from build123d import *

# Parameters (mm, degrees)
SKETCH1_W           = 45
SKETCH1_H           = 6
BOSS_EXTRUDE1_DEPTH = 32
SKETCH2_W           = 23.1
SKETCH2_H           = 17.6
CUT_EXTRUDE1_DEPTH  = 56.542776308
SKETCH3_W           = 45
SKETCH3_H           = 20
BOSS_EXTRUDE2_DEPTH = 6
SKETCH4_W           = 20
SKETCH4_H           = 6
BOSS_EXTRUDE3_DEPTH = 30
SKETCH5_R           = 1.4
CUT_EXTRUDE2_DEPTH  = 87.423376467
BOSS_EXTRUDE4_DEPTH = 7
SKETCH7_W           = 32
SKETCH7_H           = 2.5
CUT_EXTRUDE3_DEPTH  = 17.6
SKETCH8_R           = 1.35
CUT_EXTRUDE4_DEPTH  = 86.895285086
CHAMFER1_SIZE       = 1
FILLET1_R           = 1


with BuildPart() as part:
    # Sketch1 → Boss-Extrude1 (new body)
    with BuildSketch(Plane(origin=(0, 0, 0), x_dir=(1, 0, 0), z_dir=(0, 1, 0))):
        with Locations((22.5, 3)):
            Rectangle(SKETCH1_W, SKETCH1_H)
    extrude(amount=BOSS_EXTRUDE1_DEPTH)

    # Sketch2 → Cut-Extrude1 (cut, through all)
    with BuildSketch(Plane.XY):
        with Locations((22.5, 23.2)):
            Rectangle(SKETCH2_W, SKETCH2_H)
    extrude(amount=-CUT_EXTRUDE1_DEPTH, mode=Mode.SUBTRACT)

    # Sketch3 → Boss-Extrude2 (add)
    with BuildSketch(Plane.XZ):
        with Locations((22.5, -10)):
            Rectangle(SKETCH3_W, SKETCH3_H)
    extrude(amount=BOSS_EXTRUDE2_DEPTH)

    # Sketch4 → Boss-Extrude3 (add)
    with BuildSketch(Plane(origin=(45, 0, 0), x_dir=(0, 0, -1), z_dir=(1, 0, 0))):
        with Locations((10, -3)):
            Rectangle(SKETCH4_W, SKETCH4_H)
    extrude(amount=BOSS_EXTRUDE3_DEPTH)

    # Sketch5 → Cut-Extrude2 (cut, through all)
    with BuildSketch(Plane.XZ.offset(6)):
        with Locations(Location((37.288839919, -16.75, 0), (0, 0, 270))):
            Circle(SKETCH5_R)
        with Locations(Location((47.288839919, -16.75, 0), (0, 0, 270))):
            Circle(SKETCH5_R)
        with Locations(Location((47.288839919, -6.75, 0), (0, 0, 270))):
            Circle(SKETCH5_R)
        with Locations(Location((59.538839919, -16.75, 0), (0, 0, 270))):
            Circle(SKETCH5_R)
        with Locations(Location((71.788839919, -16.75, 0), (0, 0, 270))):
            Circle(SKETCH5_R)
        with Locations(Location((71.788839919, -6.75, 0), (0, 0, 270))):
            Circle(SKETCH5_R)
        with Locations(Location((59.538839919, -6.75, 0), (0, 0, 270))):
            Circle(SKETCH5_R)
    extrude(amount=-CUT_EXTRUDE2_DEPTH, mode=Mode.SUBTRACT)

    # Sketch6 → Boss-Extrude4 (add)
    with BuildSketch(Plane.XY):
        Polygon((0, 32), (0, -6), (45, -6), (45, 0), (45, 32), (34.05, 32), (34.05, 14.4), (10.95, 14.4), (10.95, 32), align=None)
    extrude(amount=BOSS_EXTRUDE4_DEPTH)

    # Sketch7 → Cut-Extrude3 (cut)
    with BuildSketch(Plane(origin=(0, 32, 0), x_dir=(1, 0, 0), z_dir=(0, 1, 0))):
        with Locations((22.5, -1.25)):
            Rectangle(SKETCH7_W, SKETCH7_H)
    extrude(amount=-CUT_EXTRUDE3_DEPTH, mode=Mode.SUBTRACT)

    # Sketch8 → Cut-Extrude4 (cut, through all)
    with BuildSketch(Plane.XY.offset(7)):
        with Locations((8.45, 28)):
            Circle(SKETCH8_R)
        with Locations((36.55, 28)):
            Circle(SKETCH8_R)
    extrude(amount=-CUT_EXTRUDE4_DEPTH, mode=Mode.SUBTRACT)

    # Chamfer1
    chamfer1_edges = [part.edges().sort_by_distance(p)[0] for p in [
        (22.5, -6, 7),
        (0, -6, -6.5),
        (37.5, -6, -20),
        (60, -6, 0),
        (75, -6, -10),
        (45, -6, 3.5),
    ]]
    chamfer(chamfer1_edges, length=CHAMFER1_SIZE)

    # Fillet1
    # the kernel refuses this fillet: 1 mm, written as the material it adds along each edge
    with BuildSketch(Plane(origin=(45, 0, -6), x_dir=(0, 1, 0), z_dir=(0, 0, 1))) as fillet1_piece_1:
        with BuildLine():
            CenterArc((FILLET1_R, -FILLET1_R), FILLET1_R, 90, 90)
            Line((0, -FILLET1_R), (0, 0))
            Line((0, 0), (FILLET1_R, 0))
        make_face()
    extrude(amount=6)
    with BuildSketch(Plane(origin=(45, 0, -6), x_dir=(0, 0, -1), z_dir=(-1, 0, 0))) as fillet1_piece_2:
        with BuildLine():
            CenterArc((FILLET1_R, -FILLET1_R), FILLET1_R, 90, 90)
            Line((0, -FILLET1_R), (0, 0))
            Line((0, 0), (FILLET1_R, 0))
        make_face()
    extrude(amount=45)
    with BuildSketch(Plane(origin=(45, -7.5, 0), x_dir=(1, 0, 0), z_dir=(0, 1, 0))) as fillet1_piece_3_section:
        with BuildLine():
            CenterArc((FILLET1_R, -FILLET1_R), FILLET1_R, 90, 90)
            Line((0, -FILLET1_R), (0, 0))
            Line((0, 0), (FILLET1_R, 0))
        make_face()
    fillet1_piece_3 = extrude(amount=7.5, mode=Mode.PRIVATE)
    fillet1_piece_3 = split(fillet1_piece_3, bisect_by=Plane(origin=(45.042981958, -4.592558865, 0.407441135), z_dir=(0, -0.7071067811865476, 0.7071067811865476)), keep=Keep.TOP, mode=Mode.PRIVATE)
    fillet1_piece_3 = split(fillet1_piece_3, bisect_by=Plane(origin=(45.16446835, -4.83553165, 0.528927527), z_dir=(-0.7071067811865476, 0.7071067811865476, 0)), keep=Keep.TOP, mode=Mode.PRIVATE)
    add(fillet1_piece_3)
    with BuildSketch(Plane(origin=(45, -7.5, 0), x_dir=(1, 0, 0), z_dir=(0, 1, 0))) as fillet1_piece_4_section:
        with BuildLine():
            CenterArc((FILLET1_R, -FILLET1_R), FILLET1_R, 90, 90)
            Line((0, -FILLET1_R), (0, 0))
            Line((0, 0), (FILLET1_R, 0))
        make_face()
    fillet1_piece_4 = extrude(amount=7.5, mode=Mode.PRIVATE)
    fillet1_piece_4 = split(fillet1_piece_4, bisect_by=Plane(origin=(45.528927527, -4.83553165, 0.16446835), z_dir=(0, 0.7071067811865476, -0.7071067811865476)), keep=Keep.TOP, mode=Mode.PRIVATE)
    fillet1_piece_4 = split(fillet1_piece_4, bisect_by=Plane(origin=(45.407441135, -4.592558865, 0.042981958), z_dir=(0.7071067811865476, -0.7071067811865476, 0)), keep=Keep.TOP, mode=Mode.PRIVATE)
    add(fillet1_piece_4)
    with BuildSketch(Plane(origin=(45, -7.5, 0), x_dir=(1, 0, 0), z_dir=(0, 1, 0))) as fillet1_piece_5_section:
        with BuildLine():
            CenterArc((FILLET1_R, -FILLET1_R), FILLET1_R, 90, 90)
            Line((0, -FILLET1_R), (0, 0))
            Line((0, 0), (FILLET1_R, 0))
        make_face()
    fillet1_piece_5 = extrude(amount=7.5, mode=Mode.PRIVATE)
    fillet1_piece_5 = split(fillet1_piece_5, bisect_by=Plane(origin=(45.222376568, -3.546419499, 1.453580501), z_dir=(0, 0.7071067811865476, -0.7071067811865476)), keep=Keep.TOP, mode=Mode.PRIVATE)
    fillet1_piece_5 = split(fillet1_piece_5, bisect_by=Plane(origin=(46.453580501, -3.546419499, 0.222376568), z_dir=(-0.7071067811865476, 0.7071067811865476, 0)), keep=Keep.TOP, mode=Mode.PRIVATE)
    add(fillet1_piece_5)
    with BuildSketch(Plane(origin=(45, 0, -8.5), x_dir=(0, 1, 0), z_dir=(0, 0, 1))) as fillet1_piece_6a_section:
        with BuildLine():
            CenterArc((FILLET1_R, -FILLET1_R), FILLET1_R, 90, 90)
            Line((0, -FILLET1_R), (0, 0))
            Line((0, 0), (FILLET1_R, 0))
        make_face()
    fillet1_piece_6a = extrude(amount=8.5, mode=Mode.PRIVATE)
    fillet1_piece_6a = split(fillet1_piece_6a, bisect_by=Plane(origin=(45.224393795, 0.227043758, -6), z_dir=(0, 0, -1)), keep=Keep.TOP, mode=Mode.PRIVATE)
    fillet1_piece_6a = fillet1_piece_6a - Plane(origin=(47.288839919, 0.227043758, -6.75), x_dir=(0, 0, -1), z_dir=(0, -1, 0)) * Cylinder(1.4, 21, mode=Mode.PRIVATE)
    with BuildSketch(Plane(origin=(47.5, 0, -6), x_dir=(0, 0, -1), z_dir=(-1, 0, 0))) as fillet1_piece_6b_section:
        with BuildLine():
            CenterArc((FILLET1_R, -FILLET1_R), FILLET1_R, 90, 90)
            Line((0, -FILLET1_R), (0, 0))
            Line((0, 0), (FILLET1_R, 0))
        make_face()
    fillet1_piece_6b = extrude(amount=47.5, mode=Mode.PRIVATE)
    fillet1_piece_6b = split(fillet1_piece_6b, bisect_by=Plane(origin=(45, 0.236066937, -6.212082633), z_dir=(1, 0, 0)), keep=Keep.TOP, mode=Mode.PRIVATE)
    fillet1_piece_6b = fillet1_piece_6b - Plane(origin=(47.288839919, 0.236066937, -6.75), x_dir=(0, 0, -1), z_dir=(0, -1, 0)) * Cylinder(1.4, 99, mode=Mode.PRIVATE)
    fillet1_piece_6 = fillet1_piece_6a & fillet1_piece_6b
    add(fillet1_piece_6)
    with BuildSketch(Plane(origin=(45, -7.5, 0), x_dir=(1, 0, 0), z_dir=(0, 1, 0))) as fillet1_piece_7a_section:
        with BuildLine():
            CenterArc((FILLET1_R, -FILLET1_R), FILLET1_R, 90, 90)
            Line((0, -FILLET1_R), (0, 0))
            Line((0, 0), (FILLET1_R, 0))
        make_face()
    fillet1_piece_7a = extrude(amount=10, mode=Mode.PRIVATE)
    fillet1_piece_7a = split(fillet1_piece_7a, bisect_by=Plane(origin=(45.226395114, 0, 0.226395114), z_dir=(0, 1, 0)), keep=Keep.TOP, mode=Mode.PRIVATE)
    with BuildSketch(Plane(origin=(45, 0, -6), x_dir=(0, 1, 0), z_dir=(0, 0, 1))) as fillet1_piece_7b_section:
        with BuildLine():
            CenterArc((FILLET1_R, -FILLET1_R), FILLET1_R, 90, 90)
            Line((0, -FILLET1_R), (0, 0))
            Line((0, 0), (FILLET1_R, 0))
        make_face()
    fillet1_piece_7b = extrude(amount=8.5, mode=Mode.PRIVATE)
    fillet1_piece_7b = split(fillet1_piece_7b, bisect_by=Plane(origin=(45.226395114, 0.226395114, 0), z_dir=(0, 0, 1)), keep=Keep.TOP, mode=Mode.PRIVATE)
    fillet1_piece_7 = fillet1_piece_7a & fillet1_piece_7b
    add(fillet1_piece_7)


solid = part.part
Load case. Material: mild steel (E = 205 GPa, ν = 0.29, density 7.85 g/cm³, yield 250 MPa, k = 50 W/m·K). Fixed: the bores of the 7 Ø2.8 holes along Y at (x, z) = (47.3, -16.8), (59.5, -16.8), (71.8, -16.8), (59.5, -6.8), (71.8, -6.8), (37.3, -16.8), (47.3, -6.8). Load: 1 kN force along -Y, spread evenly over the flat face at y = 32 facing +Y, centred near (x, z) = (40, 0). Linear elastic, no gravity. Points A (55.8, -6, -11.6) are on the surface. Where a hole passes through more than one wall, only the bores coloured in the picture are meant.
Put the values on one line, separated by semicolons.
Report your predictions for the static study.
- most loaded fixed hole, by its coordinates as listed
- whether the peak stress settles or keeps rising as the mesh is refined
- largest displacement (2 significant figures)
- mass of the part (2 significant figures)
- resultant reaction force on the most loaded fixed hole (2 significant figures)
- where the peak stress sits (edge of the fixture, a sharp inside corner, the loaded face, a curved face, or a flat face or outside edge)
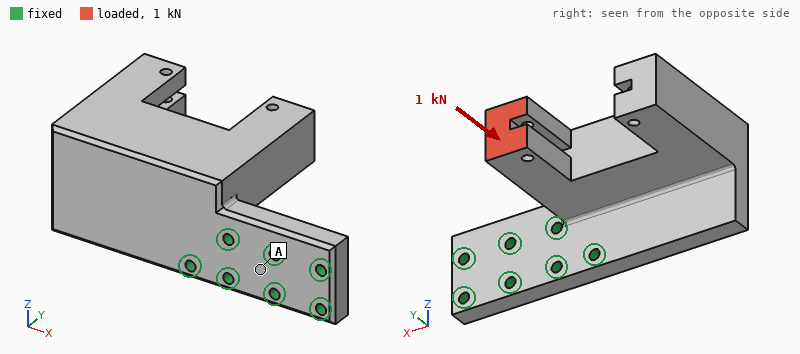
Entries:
(47.3, -6.8); keeps rising; 33 µm; 180 g; 1.0 kN; edge of the fixture
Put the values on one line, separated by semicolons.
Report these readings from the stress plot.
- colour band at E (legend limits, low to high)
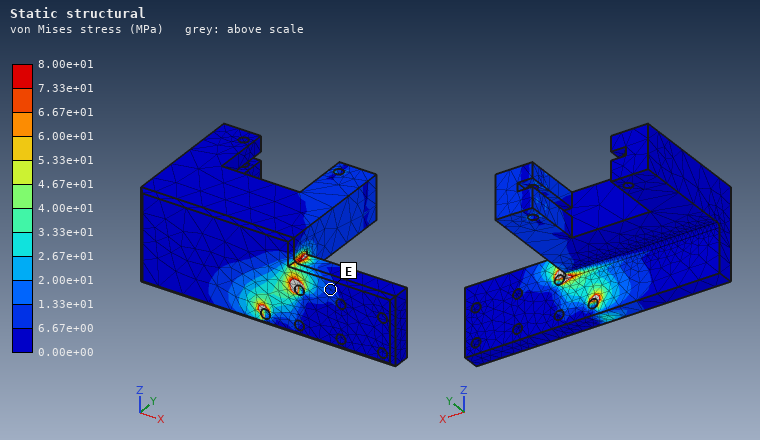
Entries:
6.67e+00 to 1.33e+01 MPa
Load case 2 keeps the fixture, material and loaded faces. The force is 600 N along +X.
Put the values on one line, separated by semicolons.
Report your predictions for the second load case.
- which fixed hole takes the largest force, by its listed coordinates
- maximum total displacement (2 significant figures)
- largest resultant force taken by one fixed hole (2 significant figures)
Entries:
(37.3, -16.8); 74 µm; 1.0 kN
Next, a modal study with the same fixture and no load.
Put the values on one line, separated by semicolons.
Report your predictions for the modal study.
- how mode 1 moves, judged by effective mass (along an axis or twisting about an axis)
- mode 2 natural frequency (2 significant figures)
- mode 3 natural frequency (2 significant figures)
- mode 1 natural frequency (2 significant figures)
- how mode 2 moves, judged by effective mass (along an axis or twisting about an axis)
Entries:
along Y; 3300 Hz; 5700 Hz; 1600 Hz; along Z
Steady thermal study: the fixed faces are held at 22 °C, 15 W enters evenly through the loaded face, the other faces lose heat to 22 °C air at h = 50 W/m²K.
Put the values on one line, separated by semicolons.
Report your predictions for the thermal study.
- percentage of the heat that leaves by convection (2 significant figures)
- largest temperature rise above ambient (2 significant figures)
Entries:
39 %; 69 K
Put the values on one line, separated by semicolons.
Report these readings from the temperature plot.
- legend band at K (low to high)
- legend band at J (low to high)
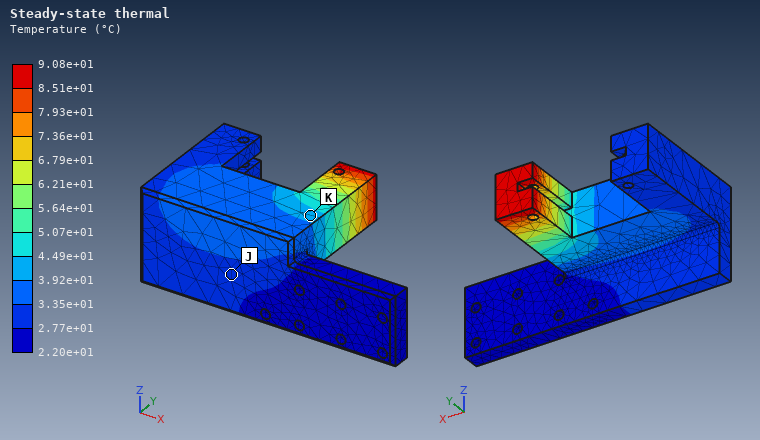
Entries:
3.92e+01 to 4.49e+01 °C; 2.77e+01 to 3.35e+01 °C
